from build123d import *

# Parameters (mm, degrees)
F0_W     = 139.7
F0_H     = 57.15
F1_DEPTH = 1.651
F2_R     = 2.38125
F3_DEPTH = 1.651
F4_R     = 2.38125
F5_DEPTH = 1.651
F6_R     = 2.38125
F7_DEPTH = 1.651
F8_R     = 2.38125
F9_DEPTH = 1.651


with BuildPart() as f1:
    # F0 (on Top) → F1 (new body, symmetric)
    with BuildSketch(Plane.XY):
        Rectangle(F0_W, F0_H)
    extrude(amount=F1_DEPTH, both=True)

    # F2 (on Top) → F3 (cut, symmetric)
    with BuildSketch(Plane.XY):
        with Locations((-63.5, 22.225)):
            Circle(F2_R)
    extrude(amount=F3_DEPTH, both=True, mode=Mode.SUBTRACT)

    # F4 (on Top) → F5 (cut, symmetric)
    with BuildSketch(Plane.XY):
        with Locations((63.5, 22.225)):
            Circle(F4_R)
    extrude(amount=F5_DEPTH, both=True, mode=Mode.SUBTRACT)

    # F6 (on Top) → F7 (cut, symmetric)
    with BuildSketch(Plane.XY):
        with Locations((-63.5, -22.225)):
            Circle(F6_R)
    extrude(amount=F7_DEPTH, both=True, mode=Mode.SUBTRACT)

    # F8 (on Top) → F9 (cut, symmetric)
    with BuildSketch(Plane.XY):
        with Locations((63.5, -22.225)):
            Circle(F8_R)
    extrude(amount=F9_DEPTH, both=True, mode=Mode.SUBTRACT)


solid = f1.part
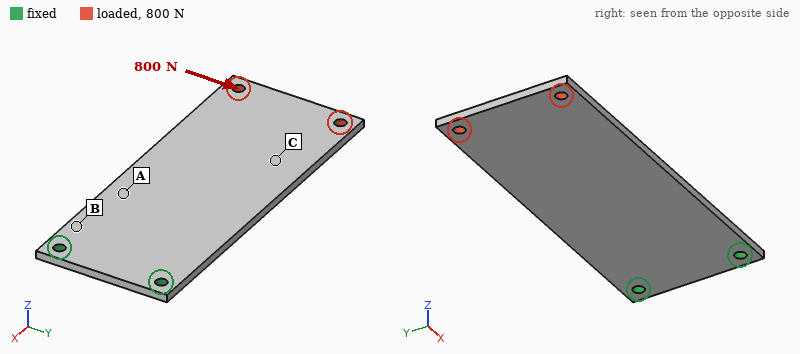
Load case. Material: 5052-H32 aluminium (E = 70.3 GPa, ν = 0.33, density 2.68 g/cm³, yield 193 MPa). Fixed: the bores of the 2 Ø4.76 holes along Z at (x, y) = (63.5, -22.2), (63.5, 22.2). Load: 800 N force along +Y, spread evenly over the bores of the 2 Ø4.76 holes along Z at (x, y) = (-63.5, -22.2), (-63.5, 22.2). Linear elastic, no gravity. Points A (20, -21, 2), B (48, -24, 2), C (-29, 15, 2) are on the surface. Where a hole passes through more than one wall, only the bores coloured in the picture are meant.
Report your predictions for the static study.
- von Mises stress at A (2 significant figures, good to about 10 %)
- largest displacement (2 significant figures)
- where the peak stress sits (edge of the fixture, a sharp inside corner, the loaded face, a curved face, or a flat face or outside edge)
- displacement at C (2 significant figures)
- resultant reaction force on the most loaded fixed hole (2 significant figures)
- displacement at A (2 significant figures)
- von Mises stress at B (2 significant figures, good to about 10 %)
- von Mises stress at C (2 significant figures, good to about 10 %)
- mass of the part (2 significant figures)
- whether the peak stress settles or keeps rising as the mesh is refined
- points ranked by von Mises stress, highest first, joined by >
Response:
28 MPa
0.20 mm
edge of the fixture
0.12 mm
2.3 kN
0.041 mm
44 MPa
11 MPa
70 g
keeps rising
B > A > C
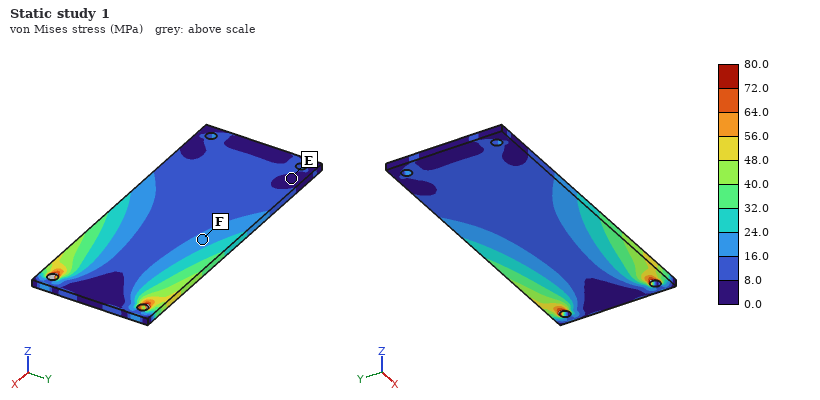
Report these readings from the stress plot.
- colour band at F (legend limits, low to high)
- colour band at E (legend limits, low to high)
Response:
16.0 to 24.0 MPa
0.0 to 8.0 MPa
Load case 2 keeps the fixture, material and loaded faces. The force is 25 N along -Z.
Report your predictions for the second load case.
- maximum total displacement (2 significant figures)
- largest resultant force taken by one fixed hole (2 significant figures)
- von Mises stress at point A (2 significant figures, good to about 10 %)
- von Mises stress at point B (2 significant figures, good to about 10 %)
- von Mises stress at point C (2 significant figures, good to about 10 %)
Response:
1.6 mm
13 N
20 MPa
29 MPa
8.4 MPa
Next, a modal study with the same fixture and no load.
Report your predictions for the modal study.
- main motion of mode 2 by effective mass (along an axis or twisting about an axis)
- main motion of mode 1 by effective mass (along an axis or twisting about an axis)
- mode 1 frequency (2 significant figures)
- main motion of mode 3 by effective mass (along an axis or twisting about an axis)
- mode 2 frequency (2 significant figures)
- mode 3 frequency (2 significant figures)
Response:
twisting about X
along Z
150 Hz
along Z
760 Hz
950 Hz
